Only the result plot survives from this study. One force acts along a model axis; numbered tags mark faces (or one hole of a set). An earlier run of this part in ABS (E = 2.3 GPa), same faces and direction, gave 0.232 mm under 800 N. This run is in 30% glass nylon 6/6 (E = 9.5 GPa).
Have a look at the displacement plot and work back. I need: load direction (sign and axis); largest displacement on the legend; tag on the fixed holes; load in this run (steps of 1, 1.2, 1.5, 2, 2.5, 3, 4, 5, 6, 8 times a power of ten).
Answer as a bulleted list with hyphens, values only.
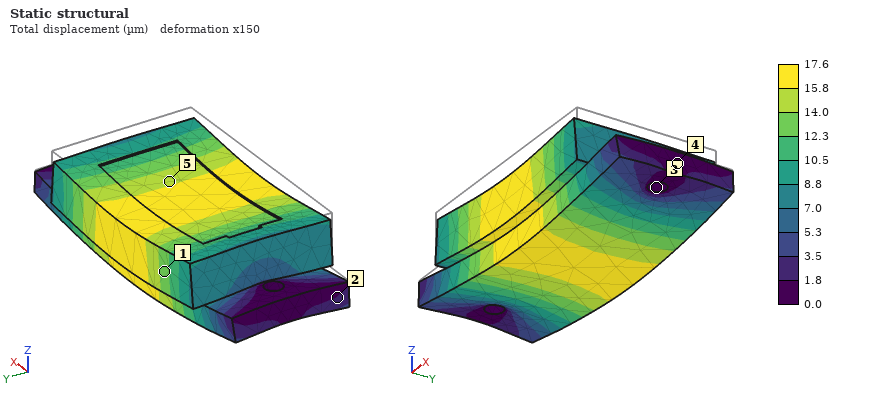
- -Z
- 17.6 µm
- 3
- 250 N
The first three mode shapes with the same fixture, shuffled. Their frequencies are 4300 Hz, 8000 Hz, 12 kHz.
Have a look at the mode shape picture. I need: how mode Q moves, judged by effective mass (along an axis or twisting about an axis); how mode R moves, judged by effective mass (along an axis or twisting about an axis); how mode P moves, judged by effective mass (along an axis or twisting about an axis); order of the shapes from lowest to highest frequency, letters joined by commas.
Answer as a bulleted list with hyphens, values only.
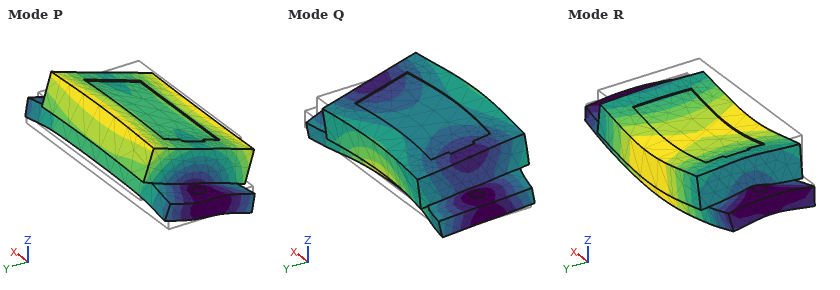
- along Y
- along Z
- along Y
- P, R, Q
